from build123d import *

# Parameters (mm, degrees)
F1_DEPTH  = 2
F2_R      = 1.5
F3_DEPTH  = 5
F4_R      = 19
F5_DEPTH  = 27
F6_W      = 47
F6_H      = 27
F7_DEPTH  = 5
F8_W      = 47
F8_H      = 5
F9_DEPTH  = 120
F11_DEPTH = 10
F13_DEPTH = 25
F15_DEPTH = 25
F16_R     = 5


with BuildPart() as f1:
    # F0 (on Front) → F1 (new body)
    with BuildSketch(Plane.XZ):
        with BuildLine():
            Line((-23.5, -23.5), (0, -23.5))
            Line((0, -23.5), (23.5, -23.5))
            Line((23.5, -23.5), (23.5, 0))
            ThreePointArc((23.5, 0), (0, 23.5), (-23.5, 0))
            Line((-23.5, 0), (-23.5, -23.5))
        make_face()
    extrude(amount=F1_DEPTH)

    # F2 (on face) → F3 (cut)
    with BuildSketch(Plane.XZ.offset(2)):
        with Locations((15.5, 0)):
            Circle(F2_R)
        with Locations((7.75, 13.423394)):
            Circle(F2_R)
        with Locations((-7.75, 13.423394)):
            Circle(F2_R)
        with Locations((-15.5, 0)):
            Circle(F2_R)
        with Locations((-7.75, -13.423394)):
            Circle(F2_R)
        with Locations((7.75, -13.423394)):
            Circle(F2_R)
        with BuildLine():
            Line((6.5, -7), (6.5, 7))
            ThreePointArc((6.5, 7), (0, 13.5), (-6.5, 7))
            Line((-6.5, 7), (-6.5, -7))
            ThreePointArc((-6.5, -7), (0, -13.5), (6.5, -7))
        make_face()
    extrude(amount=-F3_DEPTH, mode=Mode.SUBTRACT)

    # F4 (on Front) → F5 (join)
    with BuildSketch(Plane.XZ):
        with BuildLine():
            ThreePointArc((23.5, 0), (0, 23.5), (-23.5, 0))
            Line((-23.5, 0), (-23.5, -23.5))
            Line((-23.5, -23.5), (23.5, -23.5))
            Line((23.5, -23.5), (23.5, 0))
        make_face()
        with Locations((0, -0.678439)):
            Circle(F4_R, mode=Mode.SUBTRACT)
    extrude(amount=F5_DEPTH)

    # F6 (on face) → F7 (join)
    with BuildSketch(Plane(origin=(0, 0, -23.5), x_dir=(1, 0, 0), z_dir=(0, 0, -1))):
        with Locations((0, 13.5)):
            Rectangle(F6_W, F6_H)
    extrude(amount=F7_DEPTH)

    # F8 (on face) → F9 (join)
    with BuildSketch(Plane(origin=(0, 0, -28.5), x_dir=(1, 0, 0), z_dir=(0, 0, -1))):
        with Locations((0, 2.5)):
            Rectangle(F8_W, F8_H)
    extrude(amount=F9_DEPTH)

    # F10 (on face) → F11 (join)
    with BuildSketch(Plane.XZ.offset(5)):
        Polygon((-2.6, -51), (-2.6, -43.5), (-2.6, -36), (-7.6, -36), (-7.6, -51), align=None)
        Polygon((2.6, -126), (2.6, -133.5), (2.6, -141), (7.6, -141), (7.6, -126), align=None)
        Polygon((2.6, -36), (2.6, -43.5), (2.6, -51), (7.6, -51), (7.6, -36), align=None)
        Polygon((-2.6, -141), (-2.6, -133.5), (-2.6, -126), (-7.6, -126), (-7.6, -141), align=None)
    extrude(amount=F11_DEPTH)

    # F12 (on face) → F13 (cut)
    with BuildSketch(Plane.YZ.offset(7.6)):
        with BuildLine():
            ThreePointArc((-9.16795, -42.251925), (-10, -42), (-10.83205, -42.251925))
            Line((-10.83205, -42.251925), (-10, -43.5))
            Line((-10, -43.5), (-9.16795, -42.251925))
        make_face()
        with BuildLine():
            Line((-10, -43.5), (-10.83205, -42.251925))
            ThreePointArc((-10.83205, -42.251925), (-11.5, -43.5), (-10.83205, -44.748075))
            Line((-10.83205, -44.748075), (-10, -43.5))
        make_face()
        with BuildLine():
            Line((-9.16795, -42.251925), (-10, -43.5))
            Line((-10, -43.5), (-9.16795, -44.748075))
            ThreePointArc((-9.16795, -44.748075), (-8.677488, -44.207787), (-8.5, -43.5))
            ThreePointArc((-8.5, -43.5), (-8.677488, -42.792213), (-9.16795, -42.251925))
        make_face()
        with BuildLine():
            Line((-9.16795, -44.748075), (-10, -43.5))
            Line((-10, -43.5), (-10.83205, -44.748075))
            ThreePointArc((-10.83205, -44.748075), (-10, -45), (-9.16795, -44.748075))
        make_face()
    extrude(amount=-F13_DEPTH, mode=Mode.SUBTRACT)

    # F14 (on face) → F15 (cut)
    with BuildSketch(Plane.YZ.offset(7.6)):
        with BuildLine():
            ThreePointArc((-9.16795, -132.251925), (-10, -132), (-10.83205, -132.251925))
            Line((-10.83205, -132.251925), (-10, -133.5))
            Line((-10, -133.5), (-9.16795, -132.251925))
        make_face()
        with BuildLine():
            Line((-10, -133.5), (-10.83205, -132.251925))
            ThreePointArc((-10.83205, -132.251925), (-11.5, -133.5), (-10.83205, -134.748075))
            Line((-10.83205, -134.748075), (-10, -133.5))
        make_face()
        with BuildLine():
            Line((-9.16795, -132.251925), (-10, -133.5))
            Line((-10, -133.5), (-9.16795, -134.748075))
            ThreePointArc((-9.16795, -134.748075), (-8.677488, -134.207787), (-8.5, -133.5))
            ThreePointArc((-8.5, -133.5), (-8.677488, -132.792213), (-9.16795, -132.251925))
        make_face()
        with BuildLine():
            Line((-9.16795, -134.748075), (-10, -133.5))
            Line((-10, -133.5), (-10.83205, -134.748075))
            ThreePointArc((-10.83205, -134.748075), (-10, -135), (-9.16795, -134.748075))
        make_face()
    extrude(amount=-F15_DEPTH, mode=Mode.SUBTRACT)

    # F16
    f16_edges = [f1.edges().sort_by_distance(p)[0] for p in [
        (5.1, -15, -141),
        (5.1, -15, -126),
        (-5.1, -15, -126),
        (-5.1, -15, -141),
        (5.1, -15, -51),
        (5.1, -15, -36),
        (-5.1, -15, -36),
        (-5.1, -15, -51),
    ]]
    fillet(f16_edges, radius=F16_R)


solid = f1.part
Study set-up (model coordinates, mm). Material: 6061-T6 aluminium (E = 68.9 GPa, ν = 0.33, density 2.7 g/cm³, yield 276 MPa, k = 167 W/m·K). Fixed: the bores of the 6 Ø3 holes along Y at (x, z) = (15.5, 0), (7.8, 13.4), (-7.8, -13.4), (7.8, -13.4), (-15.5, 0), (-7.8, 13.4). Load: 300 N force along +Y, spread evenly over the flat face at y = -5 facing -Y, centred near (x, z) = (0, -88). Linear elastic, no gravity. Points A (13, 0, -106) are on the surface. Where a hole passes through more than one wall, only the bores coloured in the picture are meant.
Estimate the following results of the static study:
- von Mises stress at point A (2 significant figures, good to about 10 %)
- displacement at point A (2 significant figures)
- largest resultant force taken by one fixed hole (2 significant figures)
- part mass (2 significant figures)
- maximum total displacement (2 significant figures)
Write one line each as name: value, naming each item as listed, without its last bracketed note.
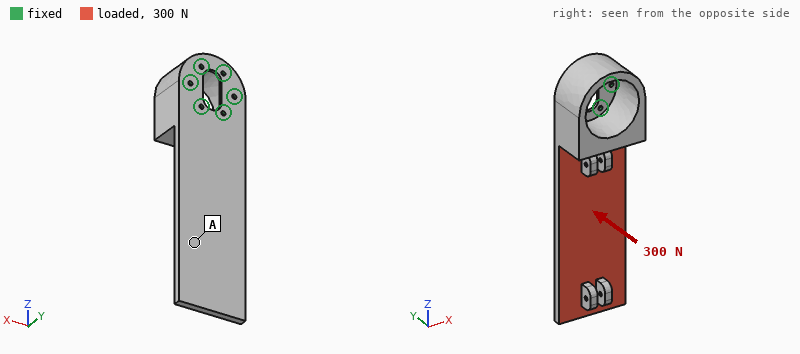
von Mises stress at point A: 12 MPa
displacement at point A: 1.1 mm
largest resultant force taken by one fixed hole: 550 N
part mass: 170 g
maximum total displacement: 2.0 mm
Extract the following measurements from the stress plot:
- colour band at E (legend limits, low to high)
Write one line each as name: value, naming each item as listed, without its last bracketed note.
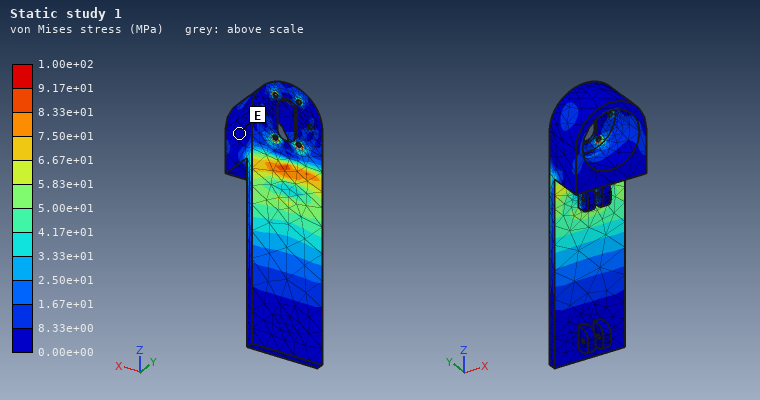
colour band at E: 0.00e+00 to 8.33e+00 MPa
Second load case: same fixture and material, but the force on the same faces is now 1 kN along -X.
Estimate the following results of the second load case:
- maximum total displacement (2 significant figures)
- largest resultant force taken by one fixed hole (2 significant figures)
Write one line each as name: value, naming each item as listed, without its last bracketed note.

maximum total displacement: 0.21 mm
largest resultant force taken by one fixed hole: 1.3 kN
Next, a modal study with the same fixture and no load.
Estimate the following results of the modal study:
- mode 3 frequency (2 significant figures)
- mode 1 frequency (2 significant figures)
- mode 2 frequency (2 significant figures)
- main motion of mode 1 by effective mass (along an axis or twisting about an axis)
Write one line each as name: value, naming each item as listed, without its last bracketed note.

mode 3 frequency: 1500 Hz
mode 1 frequency: 260 Hz
mode 2 frequency: 1400 Hz
main motion of mode 1 by effective mass: along Y
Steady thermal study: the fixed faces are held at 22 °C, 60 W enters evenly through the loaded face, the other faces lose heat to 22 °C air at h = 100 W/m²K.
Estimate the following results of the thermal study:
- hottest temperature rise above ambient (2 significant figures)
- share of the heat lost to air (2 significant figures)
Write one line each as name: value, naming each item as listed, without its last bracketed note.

hottest temperature rise above ambient: 45 K
share of the heat lost to air: 62 %
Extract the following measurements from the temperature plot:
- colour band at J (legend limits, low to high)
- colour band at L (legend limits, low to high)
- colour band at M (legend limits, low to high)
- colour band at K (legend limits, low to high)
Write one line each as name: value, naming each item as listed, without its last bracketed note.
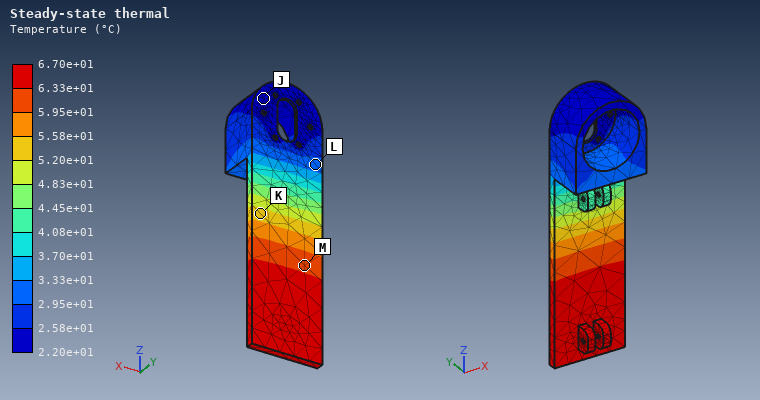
colour band at J: 2.20e+01 to 2.58e+01 °C
colour band at L: 2.95e+01 to 3.33e+01 °C
colour band at M: 5.95e+01 to 6.33e+01 °C
colour band at K: 5.20e+01 to 5.58e+01 °C
